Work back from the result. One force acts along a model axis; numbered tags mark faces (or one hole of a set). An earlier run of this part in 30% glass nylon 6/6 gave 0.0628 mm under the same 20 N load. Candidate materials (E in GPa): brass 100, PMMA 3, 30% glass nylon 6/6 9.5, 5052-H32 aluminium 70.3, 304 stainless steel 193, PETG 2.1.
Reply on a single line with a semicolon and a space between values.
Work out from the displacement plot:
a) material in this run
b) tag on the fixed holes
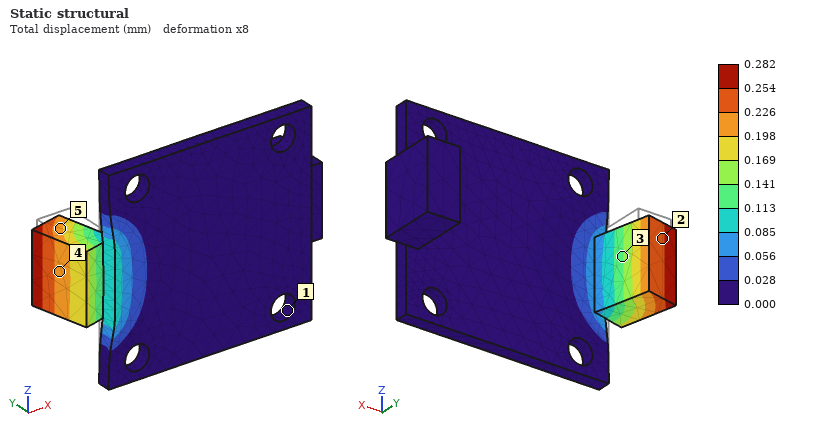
PETG; 1
